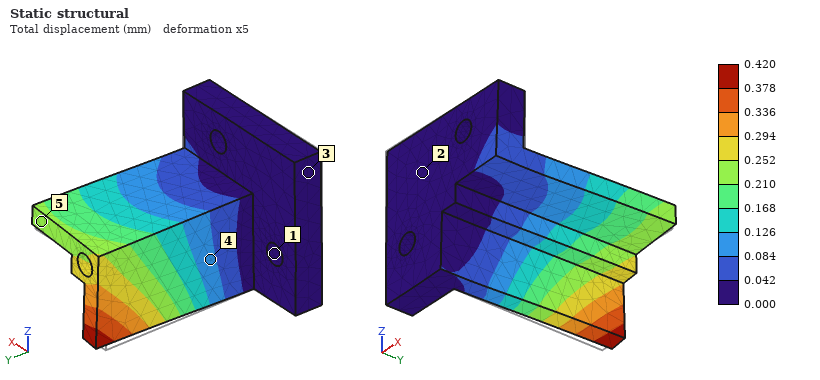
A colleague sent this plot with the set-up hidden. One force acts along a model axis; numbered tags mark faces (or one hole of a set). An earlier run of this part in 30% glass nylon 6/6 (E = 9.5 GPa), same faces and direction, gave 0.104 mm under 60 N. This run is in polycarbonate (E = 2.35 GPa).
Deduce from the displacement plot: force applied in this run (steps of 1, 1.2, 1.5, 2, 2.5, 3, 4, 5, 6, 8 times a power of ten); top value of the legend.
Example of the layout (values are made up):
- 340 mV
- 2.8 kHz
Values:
- 60 N
- 0.420 mm
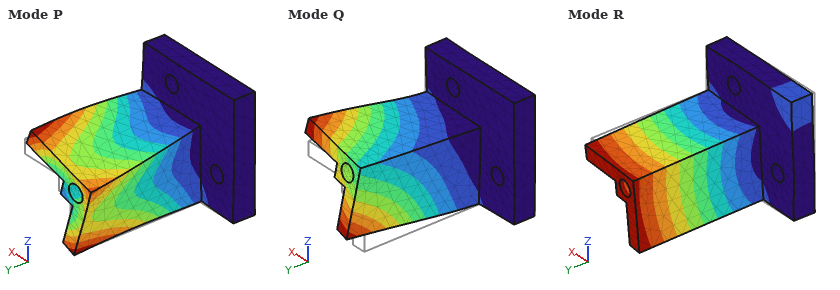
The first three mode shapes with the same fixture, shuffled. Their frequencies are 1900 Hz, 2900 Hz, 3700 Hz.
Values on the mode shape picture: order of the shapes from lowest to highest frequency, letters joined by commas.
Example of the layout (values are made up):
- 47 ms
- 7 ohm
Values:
- R, Q, P
